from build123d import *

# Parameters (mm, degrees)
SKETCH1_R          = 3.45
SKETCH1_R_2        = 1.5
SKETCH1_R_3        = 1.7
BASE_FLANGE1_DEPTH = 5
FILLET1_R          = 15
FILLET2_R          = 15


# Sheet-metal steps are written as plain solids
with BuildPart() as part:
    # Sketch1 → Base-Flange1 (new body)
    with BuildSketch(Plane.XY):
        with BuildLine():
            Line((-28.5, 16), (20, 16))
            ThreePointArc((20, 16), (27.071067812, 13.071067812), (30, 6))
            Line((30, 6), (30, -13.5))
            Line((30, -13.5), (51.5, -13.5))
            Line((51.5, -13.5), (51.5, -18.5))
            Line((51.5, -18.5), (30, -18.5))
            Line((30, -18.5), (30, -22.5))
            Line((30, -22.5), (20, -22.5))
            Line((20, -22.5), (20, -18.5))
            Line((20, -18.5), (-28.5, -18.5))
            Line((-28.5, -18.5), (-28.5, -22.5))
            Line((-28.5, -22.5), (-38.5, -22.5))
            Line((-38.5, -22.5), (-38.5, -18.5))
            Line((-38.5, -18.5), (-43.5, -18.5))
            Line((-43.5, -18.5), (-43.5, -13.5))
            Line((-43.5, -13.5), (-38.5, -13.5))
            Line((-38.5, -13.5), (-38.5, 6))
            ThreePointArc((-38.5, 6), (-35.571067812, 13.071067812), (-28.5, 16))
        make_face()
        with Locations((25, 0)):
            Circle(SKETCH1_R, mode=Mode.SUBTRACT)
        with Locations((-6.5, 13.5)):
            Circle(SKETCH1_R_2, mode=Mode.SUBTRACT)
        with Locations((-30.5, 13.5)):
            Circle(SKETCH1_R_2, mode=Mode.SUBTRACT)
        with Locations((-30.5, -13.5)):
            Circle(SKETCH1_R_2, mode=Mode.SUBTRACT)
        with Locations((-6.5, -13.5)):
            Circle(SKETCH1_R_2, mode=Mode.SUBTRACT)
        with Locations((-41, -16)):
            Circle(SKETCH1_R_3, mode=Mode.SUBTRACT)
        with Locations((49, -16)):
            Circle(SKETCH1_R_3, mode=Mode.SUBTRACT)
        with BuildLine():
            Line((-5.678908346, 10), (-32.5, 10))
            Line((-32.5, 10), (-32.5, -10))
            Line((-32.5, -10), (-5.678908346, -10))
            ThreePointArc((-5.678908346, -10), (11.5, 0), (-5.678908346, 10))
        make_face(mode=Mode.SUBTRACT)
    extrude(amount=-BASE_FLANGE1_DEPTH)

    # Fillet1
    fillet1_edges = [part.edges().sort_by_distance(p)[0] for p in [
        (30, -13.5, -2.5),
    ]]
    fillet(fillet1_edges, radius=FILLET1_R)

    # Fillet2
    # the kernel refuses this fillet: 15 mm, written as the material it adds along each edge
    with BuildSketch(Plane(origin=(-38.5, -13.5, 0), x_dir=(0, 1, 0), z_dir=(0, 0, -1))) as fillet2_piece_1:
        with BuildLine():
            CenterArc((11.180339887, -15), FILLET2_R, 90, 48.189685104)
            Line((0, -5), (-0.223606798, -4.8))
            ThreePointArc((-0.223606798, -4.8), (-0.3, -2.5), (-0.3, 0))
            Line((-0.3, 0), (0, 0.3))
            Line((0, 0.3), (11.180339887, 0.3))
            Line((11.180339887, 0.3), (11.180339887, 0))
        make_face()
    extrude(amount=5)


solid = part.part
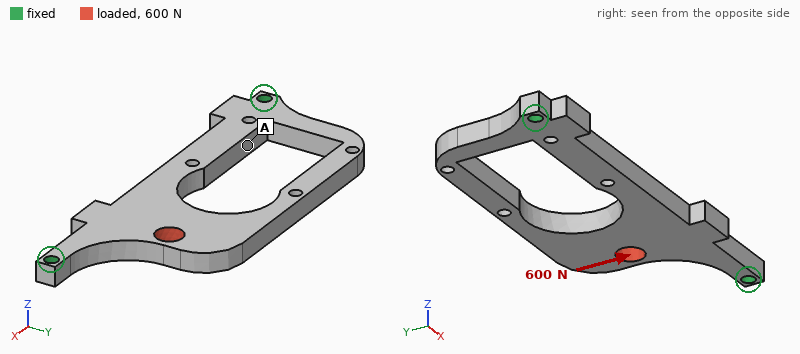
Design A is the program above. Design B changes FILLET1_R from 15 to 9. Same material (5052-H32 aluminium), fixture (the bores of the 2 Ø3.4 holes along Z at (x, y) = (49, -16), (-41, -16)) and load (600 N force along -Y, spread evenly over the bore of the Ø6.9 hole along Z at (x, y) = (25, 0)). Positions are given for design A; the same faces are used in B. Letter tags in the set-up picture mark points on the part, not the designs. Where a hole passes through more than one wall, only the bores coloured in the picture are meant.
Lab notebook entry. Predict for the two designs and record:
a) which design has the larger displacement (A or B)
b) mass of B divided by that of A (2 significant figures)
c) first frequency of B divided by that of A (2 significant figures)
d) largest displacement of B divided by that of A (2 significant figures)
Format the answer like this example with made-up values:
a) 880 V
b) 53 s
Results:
a) B
b) 0.98
c) 0.95
d) 1.2
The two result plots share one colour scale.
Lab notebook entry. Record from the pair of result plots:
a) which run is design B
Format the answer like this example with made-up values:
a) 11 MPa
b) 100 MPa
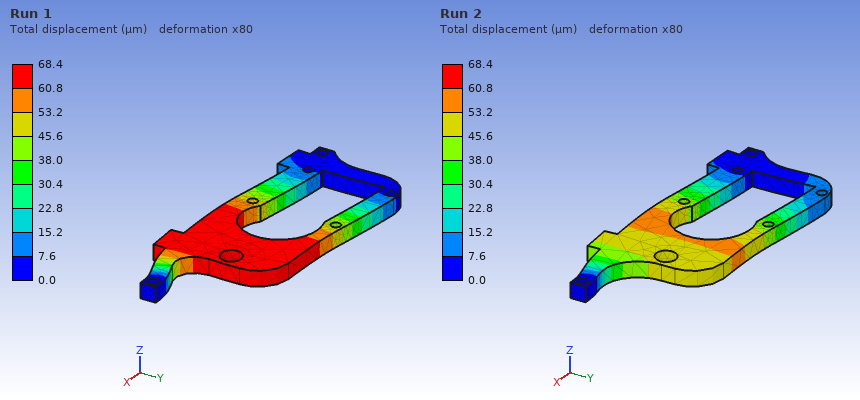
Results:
a) Run 1
